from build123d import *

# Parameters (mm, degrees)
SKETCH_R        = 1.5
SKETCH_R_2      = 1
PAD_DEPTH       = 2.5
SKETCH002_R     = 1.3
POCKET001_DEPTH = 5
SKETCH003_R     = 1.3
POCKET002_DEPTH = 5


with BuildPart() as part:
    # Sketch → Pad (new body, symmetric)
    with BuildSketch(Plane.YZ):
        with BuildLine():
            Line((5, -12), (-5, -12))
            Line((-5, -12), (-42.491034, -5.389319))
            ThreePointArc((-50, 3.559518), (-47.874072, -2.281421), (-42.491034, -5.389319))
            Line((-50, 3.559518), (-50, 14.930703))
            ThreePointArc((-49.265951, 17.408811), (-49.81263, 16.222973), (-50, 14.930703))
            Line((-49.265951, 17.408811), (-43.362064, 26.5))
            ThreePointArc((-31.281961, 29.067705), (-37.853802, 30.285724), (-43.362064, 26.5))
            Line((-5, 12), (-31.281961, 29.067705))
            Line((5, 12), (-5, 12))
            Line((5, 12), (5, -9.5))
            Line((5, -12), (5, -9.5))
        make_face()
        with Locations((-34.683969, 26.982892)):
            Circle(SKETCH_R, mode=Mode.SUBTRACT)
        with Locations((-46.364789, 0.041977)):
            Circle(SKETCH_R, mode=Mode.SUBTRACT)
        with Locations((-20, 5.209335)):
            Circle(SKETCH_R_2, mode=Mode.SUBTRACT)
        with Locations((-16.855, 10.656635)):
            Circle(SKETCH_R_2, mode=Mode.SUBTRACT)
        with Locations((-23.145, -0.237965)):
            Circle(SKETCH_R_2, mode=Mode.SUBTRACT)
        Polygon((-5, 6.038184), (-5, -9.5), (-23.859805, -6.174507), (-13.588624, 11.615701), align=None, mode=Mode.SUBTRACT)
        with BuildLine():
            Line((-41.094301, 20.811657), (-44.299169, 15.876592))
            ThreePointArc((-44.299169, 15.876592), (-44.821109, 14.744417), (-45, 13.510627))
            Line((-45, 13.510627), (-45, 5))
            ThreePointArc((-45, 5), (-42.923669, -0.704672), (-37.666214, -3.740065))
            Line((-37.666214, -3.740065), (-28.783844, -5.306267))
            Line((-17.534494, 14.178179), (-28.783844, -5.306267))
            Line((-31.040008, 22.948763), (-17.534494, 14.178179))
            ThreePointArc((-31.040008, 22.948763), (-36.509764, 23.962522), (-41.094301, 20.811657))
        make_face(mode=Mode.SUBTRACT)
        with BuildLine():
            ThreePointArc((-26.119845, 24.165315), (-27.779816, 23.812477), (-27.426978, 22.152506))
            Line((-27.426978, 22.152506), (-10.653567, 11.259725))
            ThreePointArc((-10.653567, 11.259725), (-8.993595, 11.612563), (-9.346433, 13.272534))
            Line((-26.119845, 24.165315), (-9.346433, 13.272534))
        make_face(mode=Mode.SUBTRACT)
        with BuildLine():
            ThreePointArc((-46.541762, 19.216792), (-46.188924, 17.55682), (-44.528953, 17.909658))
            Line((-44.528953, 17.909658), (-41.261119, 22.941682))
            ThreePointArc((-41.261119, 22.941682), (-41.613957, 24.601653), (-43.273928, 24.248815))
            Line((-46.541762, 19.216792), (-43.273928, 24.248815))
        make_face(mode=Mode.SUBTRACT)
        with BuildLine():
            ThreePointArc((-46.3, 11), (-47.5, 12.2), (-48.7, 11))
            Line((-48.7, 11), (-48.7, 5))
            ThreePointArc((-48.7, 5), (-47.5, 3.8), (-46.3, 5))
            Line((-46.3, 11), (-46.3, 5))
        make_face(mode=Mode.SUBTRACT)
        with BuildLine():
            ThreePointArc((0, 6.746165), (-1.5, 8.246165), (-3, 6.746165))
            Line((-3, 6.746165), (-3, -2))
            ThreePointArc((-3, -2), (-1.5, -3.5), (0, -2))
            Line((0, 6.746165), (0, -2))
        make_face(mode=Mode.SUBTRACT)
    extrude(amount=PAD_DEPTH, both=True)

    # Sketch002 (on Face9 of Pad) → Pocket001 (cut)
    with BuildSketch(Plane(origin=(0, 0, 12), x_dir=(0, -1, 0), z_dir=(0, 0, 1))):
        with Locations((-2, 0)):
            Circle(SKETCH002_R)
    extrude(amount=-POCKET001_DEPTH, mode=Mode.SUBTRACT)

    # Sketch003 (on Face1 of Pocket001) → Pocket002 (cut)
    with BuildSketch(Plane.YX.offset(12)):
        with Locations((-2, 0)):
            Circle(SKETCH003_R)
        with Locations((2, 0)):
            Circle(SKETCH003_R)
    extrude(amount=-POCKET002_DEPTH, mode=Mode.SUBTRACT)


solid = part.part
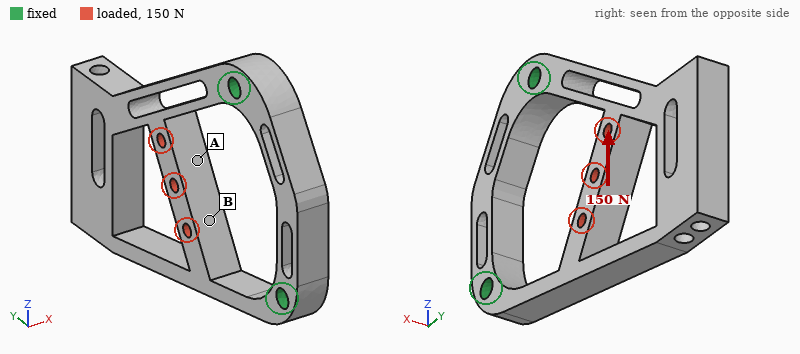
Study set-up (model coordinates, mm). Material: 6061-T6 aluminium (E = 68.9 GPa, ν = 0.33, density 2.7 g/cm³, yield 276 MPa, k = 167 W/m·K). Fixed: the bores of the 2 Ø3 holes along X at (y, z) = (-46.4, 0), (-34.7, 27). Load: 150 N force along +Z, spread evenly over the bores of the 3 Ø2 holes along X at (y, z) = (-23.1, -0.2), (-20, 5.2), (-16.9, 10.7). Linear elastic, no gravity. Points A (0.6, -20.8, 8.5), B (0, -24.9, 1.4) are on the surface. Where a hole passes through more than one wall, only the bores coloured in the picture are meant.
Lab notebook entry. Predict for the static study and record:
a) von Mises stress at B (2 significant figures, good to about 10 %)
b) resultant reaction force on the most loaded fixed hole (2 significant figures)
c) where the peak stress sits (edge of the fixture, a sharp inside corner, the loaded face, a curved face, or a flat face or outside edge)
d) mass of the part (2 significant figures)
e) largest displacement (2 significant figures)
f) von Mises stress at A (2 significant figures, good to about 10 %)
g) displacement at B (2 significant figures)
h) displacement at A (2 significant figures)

32 MPa
100 N
a curved face
8.9 g
78 µm
13 MPa
77 µm
78 µm
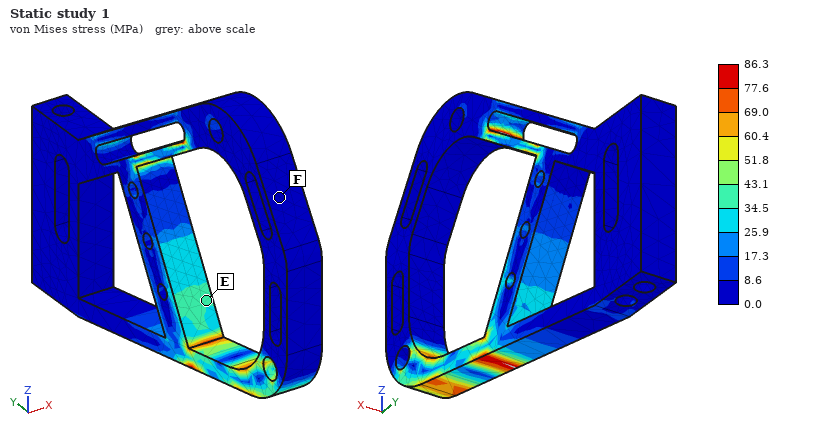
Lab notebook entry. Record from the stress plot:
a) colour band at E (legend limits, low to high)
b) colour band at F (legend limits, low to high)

34.5 to 43.1 MPa
0.0 to 8.6 MPa
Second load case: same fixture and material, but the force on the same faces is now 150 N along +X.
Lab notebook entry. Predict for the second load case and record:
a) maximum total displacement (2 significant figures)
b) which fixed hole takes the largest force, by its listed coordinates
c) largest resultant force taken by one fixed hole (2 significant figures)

0.34 mm
(-34.7, 27)
84 N
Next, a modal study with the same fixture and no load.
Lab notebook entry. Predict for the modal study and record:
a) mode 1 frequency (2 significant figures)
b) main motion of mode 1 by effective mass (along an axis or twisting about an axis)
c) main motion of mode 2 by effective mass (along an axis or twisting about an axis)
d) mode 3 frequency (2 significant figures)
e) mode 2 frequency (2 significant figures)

1200 Hz
along X
along Z
4200 Hz
3100 Hz
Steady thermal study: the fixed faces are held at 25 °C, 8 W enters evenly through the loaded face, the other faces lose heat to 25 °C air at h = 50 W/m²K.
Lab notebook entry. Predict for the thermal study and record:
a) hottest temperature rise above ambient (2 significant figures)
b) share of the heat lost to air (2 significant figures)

34 K
33 %
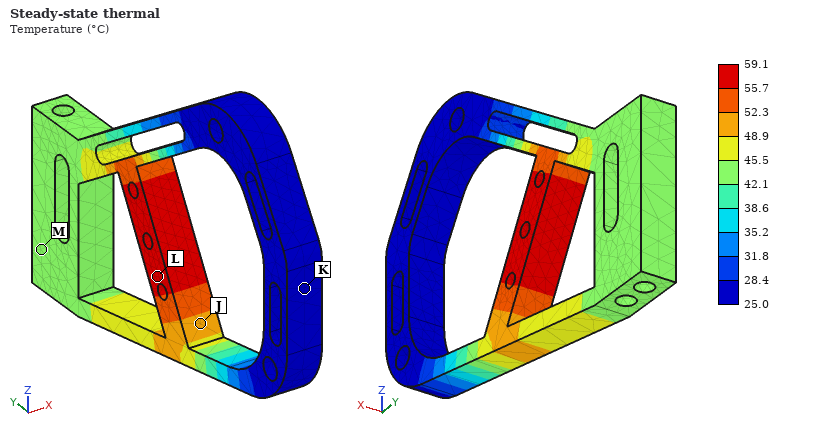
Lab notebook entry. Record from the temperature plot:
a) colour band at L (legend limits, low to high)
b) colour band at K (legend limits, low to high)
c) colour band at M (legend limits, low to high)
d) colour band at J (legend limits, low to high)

55.7 to 59.1 °C
25.0 to 28.4 °C
42.1 to 45.5 °C
48.9 to 52.3 °C
